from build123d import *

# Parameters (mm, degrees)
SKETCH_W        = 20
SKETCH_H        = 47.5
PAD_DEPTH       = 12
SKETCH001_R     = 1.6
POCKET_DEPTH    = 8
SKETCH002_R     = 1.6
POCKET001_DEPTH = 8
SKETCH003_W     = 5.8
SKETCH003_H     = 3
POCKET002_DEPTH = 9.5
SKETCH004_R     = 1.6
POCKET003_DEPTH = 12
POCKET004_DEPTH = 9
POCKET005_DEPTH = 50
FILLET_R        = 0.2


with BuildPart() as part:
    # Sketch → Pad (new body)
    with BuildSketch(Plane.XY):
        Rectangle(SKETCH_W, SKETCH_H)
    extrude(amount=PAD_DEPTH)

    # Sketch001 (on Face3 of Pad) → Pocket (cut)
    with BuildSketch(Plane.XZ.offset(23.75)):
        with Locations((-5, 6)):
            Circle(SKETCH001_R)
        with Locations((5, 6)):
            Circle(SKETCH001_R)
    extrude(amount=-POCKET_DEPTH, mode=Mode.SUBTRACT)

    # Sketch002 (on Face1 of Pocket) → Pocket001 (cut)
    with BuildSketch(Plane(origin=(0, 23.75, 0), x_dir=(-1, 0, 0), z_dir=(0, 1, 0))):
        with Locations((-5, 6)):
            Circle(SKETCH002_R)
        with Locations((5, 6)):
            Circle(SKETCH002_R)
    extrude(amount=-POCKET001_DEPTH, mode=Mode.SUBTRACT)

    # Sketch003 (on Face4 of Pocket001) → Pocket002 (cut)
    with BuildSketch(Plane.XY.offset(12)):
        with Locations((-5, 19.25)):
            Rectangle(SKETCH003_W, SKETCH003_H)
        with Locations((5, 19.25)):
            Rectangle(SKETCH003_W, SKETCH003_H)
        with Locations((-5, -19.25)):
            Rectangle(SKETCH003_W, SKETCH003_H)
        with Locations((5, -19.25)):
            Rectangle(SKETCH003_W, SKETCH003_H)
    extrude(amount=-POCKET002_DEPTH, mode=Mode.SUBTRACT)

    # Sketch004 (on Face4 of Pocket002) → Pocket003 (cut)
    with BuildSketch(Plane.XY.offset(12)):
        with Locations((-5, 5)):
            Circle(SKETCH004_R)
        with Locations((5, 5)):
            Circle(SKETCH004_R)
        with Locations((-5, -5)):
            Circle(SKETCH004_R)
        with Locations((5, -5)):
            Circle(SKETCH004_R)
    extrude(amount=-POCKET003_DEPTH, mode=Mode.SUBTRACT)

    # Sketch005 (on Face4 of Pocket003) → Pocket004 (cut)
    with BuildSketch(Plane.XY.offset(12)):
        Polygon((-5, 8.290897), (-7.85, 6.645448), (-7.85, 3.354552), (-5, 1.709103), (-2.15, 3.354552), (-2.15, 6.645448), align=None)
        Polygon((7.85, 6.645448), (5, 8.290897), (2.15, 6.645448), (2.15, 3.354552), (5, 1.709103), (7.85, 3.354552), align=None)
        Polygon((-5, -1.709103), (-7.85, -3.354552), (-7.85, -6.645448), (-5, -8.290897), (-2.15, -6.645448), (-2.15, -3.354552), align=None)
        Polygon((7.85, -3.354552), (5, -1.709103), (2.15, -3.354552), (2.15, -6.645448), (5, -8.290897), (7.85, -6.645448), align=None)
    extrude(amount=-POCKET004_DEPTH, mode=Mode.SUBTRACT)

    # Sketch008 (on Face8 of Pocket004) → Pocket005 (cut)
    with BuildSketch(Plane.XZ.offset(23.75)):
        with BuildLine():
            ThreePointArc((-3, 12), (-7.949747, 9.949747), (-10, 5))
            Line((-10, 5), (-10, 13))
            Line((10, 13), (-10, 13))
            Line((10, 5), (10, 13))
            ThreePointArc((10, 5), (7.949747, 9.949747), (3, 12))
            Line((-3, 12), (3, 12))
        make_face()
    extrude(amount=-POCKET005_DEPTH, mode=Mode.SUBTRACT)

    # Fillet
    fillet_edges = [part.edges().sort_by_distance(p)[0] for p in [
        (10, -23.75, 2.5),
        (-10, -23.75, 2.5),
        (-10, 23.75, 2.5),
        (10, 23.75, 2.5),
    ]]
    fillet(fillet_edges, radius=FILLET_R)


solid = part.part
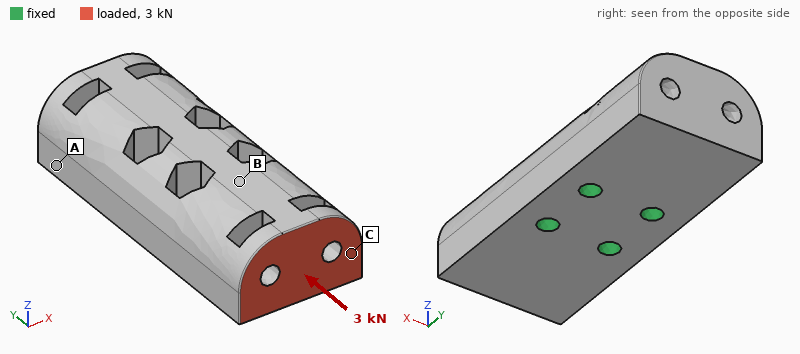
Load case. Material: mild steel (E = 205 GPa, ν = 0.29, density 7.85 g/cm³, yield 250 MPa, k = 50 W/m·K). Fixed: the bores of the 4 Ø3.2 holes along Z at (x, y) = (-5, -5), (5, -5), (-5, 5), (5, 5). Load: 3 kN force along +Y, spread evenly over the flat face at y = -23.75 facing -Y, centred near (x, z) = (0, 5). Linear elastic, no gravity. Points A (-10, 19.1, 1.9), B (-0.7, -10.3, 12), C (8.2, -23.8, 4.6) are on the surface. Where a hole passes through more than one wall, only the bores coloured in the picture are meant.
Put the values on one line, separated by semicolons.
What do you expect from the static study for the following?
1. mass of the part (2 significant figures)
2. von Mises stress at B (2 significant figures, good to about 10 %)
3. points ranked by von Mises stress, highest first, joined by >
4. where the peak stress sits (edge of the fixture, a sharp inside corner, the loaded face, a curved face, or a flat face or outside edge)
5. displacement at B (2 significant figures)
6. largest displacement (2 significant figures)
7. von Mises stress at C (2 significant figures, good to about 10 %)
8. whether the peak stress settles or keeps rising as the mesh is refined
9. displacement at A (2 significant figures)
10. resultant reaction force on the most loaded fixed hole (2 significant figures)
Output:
67 g; 32 MPa; B > C > A; edge of the fixture; 4.0 µm; 9.0 µm; 18 MPa; keeps rising; 2.3 µm; 1.1 kN
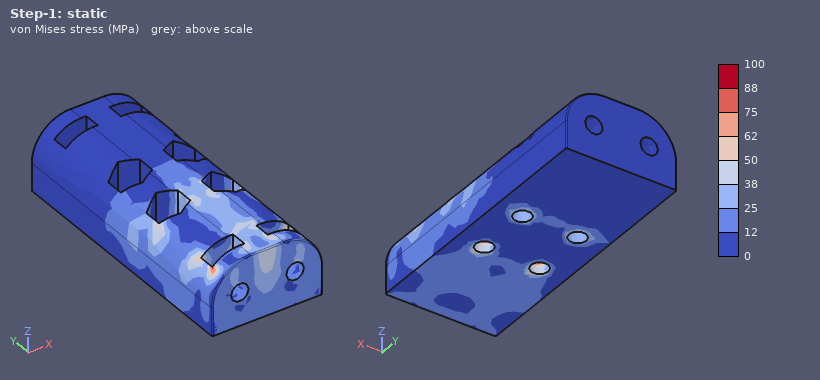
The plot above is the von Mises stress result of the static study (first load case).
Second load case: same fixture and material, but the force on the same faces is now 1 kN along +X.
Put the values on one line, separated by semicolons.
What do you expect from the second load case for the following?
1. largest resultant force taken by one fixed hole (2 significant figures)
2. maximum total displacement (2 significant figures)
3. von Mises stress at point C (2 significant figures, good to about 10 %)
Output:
1.2 kN; 7.1 µm; 14 MPa
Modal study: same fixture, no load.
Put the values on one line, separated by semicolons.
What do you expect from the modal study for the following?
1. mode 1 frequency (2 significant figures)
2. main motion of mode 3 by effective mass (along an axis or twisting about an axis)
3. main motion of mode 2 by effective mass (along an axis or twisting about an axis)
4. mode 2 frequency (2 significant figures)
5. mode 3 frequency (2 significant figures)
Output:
11 kHz; twisting about Z; along Z; 16 kHz; 20 kHz
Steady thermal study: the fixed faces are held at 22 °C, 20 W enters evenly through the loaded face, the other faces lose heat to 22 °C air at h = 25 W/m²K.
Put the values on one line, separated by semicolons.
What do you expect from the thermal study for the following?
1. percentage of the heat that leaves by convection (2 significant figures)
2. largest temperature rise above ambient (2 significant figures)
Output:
6.9 %; 56 K
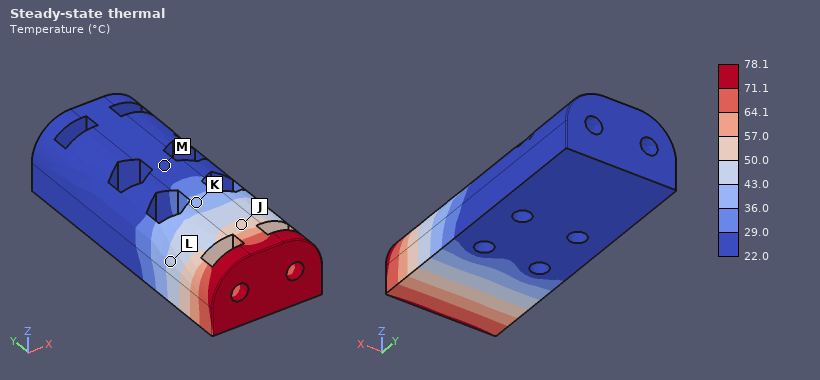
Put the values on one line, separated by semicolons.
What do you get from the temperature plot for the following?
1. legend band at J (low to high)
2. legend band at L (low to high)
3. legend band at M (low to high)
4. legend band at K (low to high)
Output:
50.0 to 57.0 °C; 43.0 to 50.0 °C; 22.0 to 29.0 °C; 36.0 to 43.0 °C
